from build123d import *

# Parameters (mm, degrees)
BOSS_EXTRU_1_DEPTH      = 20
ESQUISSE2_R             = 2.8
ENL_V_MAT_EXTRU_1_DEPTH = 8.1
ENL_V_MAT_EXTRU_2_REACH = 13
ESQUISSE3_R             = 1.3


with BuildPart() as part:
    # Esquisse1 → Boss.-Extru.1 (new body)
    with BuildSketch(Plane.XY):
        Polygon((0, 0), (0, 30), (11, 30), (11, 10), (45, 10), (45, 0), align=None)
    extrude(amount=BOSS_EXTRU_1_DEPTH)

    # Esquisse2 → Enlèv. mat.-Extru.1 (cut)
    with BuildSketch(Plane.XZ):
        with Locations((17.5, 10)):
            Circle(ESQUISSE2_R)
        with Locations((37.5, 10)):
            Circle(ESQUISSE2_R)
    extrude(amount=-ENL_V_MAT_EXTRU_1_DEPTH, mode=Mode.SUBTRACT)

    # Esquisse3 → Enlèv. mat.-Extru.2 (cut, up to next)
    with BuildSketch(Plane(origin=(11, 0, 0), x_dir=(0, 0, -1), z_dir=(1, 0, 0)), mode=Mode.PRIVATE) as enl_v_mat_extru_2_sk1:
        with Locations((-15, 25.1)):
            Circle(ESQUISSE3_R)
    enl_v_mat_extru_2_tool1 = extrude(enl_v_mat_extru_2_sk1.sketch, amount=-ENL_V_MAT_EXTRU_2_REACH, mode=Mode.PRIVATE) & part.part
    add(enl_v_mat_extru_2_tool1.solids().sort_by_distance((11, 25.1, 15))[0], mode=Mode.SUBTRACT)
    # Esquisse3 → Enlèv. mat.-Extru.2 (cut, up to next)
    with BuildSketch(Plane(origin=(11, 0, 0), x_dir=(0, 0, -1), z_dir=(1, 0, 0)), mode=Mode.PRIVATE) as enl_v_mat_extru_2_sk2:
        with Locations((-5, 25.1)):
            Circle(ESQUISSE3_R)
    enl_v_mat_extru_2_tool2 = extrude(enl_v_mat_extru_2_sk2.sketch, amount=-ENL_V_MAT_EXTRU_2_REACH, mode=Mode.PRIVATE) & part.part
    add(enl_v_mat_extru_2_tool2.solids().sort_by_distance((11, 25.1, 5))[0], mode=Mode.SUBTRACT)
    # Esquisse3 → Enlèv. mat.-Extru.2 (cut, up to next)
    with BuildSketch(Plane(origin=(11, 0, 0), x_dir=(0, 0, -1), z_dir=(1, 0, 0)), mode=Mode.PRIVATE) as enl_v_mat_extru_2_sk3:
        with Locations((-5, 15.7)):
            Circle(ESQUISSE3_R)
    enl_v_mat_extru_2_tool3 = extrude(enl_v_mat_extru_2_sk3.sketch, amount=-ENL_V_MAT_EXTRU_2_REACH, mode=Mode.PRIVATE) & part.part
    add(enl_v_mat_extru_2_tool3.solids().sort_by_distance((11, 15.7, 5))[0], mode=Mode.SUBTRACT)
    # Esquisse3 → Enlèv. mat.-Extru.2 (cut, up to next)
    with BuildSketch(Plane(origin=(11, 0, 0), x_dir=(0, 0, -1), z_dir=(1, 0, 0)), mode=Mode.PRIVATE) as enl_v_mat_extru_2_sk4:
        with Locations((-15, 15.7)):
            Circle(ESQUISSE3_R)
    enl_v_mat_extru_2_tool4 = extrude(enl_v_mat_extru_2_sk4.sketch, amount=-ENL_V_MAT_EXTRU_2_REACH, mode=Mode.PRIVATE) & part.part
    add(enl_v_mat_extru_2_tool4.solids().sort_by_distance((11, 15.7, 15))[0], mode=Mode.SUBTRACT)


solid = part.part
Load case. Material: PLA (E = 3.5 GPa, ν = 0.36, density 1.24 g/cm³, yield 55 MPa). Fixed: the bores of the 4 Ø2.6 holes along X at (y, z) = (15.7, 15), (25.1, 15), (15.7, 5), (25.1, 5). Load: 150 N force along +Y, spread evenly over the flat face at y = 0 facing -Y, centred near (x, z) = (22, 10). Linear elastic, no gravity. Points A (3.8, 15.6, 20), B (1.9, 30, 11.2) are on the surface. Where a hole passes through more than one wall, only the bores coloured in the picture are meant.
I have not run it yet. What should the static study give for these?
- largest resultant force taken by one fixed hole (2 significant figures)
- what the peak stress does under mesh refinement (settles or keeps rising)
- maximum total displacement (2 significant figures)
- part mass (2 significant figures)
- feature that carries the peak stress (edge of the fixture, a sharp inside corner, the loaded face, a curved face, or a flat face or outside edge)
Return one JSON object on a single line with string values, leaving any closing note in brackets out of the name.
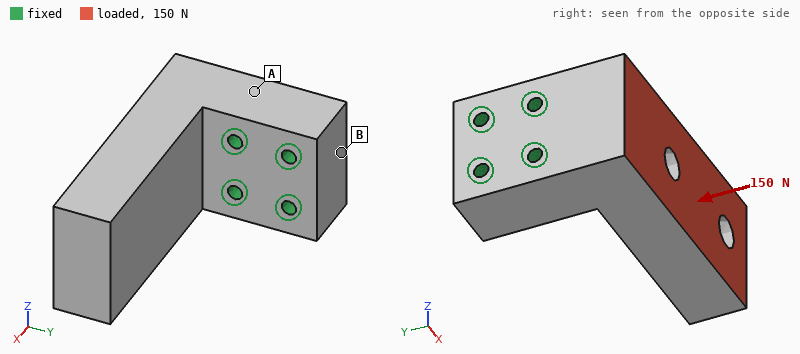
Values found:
{"largest resultant force taken by one fixed hole": "71 N", "what the peak stress does under mesh refinement": "keeps rising", "maximum total displacement": "0.28 mm", "part mass": "16 g", "feature that carries the peak stress": "edge of the fixture"}
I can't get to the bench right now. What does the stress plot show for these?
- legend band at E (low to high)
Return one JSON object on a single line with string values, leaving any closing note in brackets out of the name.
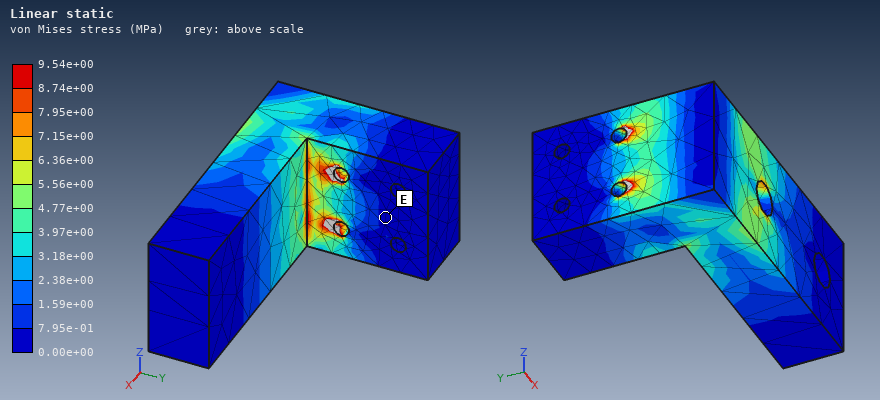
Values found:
{"legend band at E": "0.00e+00 to 7.95e-01 MPa"}
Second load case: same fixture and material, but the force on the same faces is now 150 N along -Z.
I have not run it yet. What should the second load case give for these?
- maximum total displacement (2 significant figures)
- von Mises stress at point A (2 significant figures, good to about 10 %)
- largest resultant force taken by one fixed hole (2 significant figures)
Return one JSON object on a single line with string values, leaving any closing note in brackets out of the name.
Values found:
{"maximum total displacement": "0.15 mm", "von Mises stress at point A": "3.1 MPa", "largest resultant force taken by one fixed hole": "220 N"}
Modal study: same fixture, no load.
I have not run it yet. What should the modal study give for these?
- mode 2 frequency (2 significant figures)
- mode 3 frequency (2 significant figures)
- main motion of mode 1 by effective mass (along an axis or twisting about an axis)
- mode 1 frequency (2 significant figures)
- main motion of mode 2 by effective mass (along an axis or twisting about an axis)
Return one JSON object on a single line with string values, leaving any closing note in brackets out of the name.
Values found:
{"mode 2 frequency": "1900 Hz", "mode 3 frequency": "4800 Hz", "main motion of mode 1 by effective mass": "along Y", "mode 1 frequency": "1400 Hz", "main motion of mode 2 by effective mass": "along Z"}
